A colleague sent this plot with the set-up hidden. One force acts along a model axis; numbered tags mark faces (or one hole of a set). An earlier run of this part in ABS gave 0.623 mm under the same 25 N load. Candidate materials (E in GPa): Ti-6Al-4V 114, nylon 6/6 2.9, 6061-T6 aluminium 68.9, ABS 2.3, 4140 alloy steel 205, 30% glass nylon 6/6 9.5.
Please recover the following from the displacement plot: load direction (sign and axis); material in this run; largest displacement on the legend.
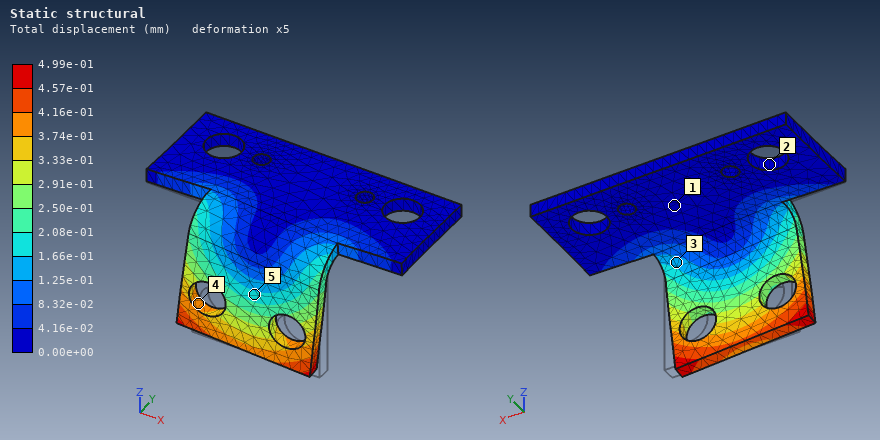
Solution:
-X
nylon 6/6
4.99e-01 mm
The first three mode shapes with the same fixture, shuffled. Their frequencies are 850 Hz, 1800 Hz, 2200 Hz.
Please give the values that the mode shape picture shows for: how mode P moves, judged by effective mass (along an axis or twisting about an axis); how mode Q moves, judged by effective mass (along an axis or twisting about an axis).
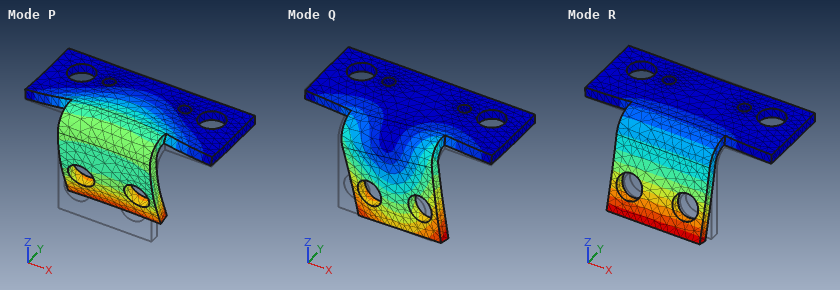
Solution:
along Z
along X
